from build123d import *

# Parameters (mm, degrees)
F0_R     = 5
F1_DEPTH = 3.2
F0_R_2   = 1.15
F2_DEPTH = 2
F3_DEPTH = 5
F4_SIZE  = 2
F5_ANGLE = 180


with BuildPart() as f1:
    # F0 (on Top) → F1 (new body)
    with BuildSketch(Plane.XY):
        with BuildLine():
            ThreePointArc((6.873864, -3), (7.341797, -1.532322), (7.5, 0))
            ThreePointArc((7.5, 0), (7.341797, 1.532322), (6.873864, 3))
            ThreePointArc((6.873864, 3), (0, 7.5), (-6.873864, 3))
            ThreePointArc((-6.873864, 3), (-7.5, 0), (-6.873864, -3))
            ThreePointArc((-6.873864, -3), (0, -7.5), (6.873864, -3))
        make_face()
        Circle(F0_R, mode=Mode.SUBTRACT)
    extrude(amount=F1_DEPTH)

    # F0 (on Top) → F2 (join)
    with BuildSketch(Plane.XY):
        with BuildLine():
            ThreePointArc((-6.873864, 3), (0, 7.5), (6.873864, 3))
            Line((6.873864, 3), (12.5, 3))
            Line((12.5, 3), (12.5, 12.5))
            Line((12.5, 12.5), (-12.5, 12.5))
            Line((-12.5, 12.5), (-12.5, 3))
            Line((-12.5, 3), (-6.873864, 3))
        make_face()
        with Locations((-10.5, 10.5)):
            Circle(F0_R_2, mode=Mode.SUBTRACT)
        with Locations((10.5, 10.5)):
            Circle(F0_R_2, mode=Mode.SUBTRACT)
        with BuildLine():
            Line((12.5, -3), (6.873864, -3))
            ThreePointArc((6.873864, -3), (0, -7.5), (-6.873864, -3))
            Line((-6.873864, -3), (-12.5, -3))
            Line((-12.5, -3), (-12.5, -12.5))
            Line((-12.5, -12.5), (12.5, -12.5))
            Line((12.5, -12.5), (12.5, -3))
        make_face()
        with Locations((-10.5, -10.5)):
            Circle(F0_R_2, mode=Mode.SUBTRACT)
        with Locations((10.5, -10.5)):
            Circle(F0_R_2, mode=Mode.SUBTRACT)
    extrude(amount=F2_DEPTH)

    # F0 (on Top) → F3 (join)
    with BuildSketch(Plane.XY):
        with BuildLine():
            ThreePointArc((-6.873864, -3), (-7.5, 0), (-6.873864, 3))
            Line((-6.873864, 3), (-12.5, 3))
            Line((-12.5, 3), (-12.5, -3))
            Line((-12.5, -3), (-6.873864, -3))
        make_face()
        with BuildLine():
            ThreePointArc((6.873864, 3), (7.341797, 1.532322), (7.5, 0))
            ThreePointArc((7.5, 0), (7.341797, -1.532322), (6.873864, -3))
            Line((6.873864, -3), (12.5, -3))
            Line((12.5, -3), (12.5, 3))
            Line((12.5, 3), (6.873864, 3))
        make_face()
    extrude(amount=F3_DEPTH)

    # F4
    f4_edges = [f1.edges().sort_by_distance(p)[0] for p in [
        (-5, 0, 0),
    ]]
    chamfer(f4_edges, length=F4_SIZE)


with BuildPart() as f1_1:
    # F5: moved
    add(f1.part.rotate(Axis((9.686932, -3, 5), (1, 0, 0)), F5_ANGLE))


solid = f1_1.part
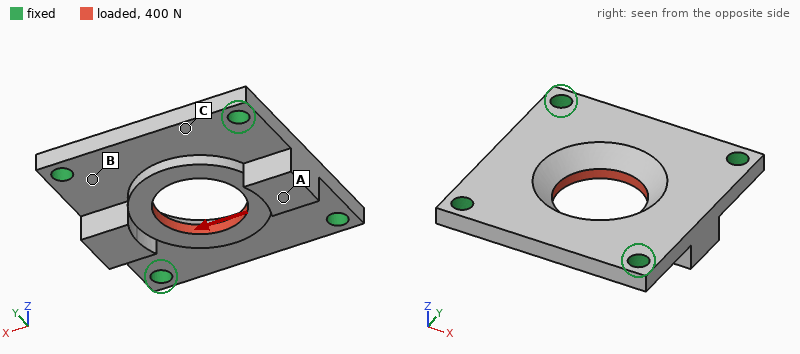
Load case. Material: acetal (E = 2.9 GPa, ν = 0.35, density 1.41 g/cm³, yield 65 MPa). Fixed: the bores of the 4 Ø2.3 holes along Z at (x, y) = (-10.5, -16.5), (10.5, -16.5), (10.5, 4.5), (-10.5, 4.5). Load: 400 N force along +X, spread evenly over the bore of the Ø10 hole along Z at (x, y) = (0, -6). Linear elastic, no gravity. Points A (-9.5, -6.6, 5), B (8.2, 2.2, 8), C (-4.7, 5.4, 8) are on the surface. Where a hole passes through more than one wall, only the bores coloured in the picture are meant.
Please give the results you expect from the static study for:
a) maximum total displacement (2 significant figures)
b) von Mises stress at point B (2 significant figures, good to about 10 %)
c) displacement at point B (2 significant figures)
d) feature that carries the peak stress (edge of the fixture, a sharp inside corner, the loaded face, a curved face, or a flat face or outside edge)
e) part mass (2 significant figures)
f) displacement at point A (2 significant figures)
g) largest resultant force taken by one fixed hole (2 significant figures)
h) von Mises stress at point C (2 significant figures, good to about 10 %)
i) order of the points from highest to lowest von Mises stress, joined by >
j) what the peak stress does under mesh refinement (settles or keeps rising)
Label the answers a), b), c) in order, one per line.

a) 87 µm
b) 12 MPa
c) 15 µm
d) edge of the fixture
e) 1.8 g
f) 75 µm
g) 110 N
h) 6.5 MPa
i) B > C > A
j) keeps rising
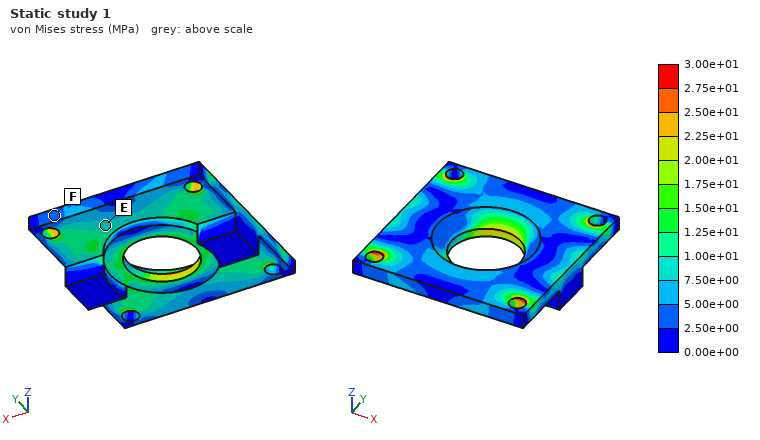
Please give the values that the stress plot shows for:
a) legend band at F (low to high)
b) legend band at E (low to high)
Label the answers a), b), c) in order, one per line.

a) 2.50e+00 to 5.00e+00 MPa
b) 7.50e+00 to 1.00e+01 MPa
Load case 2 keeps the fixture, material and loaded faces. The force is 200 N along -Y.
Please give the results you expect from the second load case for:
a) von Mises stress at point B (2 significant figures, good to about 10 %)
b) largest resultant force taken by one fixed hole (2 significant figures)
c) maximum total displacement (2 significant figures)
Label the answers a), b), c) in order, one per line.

a) 5.8 MPa
b) 55 N
c) 41 µm
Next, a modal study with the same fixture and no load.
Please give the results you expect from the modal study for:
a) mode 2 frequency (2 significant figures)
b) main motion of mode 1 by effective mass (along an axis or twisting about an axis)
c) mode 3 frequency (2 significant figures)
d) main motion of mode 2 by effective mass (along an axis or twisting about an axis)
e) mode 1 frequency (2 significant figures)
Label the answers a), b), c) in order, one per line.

a) 6600 Hz
b) along Z
c) 7300 Hz
d) twisting about Y
e) 5400 Hz
